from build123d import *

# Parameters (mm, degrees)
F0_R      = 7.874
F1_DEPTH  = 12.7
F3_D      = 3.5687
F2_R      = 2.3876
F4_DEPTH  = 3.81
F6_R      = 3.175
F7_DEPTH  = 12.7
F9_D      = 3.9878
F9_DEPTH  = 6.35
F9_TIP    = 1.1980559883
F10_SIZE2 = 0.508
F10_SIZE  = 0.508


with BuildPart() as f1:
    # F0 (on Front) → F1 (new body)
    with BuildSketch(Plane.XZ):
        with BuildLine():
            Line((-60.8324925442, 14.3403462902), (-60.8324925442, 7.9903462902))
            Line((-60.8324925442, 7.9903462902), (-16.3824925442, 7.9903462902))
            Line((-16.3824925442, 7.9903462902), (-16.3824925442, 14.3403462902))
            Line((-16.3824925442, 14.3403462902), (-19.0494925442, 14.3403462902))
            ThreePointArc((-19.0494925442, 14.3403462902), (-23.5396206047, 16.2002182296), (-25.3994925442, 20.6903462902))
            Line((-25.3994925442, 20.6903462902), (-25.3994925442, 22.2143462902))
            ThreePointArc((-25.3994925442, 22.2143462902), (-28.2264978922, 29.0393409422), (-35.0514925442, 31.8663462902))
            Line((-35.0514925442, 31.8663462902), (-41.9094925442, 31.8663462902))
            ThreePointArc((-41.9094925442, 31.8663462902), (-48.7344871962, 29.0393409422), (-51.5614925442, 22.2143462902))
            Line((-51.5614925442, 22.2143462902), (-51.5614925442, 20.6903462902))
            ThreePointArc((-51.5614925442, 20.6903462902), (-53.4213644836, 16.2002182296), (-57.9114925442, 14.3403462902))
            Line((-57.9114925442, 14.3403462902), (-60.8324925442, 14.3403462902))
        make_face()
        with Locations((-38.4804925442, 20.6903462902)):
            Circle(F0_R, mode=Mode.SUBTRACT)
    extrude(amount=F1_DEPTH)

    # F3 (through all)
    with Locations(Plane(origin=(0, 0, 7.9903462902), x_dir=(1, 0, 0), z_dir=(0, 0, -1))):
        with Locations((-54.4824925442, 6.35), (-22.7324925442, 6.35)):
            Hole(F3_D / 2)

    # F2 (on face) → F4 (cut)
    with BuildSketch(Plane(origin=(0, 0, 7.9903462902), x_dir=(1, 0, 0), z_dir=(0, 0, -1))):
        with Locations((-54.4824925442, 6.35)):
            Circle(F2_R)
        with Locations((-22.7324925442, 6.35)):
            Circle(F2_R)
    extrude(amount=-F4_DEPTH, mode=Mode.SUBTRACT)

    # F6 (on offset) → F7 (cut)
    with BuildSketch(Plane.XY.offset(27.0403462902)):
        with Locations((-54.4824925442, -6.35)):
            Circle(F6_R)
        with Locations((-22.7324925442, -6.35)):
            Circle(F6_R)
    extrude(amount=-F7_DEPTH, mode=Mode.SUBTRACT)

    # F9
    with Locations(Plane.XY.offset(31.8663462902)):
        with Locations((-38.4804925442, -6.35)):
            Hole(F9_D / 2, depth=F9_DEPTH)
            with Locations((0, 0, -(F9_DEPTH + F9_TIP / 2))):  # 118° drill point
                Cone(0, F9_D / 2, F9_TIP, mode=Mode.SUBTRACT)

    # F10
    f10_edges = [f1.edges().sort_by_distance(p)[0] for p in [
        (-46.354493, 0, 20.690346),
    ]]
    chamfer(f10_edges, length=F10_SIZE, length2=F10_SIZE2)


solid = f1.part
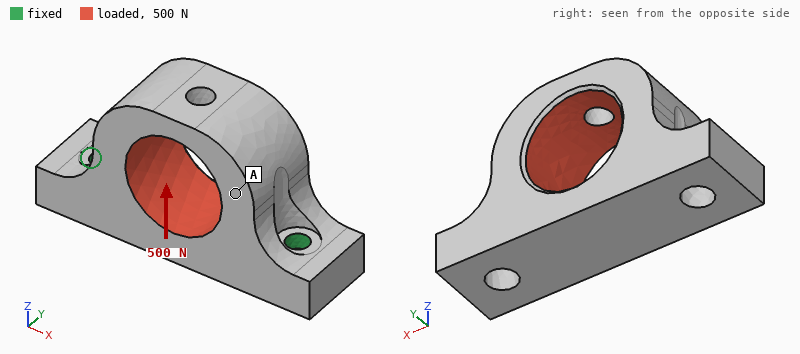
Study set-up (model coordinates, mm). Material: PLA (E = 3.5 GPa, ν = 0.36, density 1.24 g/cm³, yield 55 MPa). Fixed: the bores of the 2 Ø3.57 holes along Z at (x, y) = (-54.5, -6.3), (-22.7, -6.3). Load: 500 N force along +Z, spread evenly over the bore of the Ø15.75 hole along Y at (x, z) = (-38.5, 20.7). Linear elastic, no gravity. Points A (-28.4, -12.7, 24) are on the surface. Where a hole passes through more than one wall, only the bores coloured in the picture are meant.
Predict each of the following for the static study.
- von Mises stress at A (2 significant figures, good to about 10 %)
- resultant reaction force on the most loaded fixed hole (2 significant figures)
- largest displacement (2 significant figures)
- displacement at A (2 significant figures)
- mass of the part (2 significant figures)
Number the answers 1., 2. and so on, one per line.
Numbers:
1. 3.9 MPa
2. 250 N
3. 66 µm
4. 44 µm
5. 7.8 g
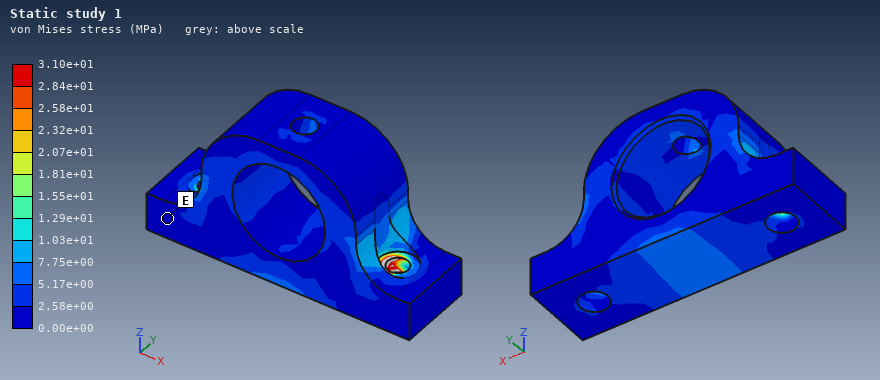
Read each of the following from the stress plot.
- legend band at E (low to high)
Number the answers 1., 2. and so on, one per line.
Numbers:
1. 0.00e+00 to 2.58e+00 MPa
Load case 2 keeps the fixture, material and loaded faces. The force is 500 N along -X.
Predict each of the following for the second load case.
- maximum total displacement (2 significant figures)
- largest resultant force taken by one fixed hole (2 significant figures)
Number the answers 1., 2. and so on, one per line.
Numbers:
1. 84 µm
2. 280 N
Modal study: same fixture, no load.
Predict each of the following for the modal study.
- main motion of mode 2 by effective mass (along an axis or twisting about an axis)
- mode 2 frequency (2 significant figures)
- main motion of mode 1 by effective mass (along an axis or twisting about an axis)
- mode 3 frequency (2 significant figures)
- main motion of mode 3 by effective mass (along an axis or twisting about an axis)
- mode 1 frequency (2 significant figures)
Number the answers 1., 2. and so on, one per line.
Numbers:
1. along X
2. 6300 Hz
3. along Y
4. 6900 Hz
5. along Z
6. 2500 Hz
